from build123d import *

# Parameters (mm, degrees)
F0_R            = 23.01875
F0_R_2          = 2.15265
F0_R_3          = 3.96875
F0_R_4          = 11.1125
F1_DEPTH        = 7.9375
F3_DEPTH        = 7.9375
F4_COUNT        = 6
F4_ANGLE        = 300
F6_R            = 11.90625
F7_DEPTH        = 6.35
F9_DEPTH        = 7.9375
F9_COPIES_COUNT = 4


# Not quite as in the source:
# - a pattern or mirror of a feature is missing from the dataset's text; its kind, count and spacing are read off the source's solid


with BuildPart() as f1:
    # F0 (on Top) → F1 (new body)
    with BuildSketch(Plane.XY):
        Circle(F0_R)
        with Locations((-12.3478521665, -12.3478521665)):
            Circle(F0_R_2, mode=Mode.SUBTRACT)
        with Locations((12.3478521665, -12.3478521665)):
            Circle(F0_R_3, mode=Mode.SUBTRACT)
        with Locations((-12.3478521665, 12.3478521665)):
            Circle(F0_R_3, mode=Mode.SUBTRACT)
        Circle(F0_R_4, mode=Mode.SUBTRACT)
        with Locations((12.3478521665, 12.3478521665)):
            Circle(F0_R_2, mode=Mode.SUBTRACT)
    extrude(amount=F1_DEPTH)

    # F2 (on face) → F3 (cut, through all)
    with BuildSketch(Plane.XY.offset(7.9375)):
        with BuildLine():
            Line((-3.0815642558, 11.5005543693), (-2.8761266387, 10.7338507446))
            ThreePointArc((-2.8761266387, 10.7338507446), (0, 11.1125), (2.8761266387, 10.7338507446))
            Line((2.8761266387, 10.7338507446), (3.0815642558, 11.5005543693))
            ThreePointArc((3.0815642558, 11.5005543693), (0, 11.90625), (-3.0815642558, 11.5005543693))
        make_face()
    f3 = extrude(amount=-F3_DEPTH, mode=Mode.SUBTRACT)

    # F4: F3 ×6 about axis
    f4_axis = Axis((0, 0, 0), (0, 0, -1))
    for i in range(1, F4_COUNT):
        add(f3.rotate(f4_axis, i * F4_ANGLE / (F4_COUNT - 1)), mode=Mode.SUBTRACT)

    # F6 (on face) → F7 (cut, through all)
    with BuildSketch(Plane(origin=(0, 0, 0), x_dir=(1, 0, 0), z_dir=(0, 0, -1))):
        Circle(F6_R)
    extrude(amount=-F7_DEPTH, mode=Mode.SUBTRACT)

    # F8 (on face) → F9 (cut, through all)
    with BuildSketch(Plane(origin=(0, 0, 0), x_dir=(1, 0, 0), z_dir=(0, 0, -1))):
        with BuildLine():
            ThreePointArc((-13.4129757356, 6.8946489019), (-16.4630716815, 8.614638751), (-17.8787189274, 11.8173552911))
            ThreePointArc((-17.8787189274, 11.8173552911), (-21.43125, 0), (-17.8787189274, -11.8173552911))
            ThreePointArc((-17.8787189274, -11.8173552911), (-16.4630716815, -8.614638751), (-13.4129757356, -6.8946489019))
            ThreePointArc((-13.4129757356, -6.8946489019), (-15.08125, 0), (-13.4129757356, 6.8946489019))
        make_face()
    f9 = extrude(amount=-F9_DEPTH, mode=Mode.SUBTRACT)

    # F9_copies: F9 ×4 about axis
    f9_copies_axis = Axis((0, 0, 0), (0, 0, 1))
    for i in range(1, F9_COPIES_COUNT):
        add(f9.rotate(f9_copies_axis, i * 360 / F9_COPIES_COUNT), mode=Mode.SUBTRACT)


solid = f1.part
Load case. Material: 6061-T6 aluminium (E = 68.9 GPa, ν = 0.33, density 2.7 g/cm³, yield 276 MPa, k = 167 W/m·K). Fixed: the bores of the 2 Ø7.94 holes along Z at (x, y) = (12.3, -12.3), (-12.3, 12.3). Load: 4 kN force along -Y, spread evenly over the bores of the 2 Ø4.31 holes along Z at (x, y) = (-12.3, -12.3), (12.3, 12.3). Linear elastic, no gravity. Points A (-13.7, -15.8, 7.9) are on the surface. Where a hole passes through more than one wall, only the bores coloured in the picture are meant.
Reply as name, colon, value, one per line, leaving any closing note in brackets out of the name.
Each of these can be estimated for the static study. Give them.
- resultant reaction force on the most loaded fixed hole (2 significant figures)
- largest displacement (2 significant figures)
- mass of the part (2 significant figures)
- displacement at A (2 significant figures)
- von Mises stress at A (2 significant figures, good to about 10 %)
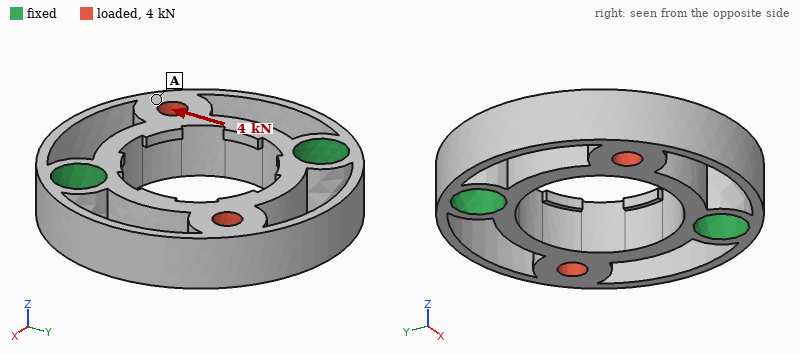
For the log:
resultant reaction force on the most loaded fixed hole: 2.0 kN
largest displacement: 36 µm
mass of the part: 14 g
displacement at A: 27 µm
von Mises stress at A: 22 MPa
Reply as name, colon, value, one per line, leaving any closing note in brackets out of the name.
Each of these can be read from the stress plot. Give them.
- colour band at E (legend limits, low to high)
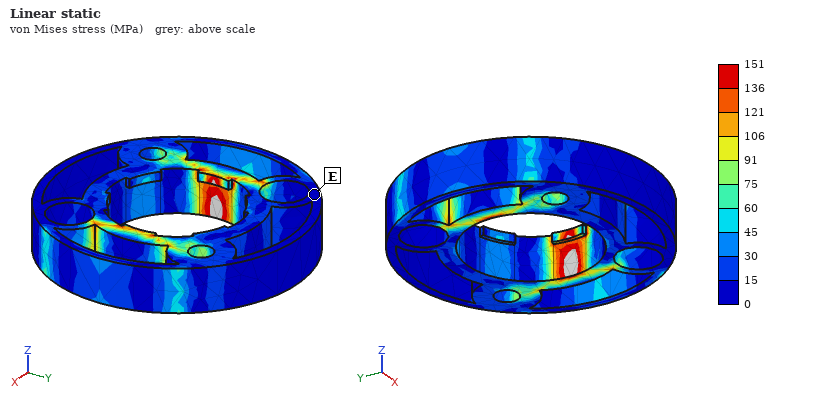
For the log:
colour band at E: 0 to 15 MPa
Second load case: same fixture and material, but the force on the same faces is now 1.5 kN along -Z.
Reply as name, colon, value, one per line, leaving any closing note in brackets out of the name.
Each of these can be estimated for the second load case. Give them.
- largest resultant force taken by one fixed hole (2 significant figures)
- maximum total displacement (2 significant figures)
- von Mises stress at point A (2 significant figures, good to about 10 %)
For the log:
largest resultant force taken by one fixed hole: 750 N
maximum total displacement: 0.11 mm
von Mises stress at point A: 32 MPa
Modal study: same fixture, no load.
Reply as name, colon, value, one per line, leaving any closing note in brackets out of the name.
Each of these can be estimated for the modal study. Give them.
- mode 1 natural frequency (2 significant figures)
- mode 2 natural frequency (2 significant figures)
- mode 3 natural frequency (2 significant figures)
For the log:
mode 1 natural frequency: 8400 Hz
mode 2 natural frequency: 8400 Hz
mode 3 natural frequency: 16 kHz
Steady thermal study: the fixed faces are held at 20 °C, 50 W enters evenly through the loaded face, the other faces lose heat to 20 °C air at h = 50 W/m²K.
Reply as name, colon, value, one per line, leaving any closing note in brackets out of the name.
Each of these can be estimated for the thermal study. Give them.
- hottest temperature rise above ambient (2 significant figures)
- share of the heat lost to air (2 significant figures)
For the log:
hottest temperature rise above ambient: 39 K
share of the heat lost to air: 8.7 %
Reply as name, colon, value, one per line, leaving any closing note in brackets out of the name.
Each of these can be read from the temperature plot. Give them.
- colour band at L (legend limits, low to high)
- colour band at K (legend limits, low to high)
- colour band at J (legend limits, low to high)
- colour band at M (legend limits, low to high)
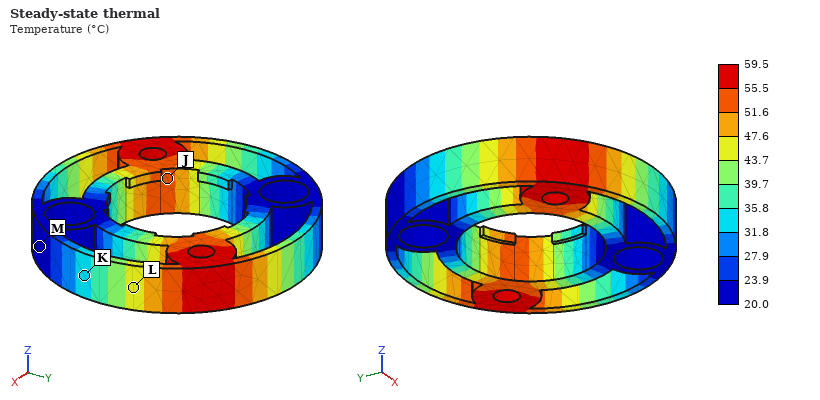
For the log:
colour band at L: 43.7 to 47.6 °C
colour band at K: 31.8 to 35.8 °C
colour band at J: 51.6 to 55.5 °C
colour band at M: 20.0 to 23.9 °C
